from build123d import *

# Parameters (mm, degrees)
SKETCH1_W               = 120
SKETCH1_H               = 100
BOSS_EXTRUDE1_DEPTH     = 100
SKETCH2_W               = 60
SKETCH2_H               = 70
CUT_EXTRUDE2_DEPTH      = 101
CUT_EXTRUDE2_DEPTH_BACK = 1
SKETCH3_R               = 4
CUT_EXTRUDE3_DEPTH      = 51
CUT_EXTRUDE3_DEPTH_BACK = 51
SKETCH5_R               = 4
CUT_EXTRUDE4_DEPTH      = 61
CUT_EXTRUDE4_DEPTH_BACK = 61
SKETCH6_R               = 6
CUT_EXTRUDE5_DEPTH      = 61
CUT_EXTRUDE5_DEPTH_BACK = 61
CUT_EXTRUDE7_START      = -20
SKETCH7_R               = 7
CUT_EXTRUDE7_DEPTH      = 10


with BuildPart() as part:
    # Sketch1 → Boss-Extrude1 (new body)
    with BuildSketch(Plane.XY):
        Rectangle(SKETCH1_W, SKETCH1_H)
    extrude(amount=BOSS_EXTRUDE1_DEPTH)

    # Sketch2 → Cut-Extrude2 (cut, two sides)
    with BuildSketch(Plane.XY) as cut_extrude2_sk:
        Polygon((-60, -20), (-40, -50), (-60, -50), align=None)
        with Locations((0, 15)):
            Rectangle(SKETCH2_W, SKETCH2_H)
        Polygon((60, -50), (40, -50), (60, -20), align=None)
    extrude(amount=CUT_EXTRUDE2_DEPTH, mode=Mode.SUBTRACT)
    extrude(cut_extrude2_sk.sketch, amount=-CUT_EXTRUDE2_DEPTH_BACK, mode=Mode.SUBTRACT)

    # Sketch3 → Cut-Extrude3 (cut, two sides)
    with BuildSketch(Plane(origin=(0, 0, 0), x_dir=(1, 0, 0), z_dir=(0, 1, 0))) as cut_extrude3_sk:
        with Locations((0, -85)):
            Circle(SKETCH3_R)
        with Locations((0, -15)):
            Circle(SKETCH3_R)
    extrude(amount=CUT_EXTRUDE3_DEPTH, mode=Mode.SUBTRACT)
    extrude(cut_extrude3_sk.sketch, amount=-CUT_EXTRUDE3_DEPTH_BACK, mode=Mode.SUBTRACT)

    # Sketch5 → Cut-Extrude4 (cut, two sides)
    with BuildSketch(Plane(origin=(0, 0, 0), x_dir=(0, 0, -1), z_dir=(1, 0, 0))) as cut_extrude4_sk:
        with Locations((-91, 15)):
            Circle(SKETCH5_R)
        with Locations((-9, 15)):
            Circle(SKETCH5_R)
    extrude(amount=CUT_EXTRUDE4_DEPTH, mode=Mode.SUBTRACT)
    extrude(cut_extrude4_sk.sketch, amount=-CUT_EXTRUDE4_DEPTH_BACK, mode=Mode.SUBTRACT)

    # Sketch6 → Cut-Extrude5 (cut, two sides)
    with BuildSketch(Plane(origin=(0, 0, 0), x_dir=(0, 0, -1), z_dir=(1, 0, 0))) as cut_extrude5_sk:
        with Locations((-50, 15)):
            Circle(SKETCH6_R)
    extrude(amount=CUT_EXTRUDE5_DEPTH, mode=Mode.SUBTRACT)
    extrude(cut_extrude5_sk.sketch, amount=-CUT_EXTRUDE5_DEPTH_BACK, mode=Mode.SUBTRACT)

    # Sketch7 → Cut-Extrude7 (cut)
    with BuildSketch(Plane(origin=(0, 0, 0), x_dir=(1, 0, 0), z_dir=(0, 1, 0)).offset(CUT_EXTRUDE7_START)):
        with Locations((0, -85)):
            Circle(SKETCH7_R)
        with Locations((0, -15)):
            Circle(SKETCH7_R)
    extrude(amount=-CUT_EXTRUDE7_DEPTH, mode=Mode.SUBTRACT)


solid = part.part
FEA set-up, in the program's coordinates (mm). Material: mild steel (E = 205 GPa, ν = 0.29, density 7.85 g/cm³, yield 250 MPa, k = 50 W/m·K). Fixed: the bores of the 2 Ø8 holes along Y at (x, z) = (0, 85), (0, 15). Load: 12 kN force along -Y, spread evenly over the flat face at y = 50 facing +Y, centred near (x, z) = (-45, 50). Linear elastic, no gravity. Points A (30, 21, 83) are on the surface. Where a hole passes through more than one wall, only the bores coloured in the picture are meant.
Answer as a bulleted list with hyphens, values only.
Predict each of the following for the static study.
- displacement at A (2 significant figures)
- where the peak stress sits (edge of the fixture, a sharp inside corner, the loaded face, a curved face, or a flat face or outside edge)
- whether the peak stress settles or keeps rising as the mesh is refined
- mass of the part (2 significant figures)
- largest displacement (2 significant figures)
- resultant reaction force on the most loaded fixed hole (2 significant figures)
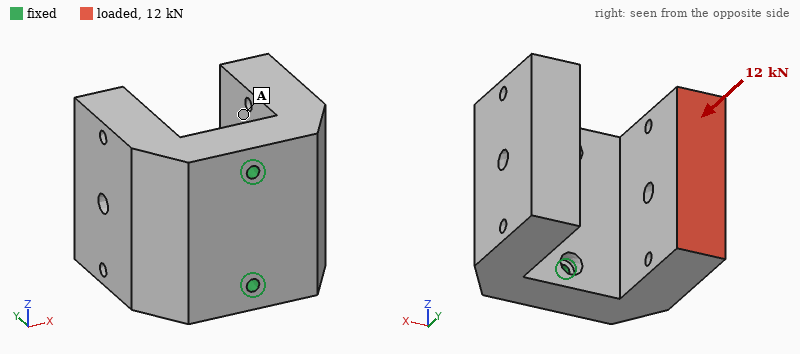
- 25 µm
- edge of the fixture
- keeps rising
- 5.5 kg
- 72 µm
- 6.1 kN
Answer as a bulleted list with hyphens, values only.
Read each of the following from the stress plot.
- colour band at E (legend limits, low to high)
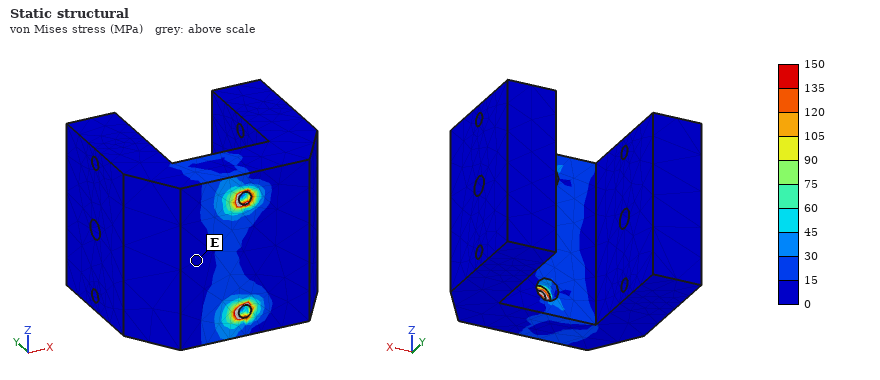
- 0 to 15 MPa
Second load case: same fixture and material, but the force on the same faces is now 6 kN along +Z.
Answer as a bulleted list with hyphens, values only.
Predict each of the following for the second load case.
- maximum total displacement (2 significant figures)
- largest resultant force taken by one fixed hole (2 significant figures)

- 29 µm
- 8.5 kN
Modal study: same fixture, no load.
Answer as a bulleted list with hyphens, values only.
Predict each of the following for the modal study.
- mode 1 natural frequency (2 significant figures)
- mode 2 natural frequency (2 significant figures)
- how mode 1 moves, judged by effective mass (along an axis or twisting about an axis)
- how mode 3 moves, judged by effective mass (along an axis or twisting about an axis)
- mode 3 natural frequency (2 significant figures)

- 1100 Hz
- 1800 Hz
- along X
- along Z
- 2700 Hz
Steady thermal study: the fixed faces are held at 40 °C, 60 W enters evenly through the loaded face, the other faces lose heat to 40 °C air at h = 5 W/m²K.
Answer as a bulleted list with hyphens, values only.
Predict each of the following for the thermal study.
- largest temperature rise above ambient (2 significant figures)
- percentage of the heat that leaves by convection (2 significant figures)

- 51 K
- 9.1 %
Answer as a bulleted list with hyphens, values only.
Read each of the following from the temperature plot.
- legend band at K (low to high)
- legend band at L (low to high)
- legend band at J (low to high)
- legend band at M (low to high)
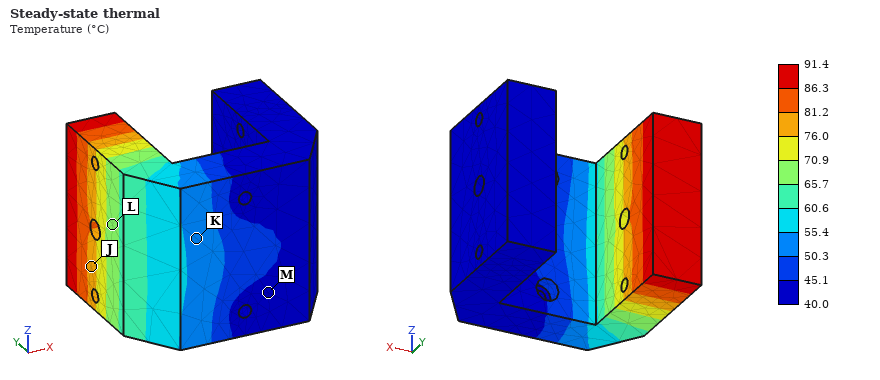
- 50.3 to 55.4 °C
- 65.7 to 70.9 °C
- 76.0 to 81.2 °C
- 40.0 to 45.1 °C
